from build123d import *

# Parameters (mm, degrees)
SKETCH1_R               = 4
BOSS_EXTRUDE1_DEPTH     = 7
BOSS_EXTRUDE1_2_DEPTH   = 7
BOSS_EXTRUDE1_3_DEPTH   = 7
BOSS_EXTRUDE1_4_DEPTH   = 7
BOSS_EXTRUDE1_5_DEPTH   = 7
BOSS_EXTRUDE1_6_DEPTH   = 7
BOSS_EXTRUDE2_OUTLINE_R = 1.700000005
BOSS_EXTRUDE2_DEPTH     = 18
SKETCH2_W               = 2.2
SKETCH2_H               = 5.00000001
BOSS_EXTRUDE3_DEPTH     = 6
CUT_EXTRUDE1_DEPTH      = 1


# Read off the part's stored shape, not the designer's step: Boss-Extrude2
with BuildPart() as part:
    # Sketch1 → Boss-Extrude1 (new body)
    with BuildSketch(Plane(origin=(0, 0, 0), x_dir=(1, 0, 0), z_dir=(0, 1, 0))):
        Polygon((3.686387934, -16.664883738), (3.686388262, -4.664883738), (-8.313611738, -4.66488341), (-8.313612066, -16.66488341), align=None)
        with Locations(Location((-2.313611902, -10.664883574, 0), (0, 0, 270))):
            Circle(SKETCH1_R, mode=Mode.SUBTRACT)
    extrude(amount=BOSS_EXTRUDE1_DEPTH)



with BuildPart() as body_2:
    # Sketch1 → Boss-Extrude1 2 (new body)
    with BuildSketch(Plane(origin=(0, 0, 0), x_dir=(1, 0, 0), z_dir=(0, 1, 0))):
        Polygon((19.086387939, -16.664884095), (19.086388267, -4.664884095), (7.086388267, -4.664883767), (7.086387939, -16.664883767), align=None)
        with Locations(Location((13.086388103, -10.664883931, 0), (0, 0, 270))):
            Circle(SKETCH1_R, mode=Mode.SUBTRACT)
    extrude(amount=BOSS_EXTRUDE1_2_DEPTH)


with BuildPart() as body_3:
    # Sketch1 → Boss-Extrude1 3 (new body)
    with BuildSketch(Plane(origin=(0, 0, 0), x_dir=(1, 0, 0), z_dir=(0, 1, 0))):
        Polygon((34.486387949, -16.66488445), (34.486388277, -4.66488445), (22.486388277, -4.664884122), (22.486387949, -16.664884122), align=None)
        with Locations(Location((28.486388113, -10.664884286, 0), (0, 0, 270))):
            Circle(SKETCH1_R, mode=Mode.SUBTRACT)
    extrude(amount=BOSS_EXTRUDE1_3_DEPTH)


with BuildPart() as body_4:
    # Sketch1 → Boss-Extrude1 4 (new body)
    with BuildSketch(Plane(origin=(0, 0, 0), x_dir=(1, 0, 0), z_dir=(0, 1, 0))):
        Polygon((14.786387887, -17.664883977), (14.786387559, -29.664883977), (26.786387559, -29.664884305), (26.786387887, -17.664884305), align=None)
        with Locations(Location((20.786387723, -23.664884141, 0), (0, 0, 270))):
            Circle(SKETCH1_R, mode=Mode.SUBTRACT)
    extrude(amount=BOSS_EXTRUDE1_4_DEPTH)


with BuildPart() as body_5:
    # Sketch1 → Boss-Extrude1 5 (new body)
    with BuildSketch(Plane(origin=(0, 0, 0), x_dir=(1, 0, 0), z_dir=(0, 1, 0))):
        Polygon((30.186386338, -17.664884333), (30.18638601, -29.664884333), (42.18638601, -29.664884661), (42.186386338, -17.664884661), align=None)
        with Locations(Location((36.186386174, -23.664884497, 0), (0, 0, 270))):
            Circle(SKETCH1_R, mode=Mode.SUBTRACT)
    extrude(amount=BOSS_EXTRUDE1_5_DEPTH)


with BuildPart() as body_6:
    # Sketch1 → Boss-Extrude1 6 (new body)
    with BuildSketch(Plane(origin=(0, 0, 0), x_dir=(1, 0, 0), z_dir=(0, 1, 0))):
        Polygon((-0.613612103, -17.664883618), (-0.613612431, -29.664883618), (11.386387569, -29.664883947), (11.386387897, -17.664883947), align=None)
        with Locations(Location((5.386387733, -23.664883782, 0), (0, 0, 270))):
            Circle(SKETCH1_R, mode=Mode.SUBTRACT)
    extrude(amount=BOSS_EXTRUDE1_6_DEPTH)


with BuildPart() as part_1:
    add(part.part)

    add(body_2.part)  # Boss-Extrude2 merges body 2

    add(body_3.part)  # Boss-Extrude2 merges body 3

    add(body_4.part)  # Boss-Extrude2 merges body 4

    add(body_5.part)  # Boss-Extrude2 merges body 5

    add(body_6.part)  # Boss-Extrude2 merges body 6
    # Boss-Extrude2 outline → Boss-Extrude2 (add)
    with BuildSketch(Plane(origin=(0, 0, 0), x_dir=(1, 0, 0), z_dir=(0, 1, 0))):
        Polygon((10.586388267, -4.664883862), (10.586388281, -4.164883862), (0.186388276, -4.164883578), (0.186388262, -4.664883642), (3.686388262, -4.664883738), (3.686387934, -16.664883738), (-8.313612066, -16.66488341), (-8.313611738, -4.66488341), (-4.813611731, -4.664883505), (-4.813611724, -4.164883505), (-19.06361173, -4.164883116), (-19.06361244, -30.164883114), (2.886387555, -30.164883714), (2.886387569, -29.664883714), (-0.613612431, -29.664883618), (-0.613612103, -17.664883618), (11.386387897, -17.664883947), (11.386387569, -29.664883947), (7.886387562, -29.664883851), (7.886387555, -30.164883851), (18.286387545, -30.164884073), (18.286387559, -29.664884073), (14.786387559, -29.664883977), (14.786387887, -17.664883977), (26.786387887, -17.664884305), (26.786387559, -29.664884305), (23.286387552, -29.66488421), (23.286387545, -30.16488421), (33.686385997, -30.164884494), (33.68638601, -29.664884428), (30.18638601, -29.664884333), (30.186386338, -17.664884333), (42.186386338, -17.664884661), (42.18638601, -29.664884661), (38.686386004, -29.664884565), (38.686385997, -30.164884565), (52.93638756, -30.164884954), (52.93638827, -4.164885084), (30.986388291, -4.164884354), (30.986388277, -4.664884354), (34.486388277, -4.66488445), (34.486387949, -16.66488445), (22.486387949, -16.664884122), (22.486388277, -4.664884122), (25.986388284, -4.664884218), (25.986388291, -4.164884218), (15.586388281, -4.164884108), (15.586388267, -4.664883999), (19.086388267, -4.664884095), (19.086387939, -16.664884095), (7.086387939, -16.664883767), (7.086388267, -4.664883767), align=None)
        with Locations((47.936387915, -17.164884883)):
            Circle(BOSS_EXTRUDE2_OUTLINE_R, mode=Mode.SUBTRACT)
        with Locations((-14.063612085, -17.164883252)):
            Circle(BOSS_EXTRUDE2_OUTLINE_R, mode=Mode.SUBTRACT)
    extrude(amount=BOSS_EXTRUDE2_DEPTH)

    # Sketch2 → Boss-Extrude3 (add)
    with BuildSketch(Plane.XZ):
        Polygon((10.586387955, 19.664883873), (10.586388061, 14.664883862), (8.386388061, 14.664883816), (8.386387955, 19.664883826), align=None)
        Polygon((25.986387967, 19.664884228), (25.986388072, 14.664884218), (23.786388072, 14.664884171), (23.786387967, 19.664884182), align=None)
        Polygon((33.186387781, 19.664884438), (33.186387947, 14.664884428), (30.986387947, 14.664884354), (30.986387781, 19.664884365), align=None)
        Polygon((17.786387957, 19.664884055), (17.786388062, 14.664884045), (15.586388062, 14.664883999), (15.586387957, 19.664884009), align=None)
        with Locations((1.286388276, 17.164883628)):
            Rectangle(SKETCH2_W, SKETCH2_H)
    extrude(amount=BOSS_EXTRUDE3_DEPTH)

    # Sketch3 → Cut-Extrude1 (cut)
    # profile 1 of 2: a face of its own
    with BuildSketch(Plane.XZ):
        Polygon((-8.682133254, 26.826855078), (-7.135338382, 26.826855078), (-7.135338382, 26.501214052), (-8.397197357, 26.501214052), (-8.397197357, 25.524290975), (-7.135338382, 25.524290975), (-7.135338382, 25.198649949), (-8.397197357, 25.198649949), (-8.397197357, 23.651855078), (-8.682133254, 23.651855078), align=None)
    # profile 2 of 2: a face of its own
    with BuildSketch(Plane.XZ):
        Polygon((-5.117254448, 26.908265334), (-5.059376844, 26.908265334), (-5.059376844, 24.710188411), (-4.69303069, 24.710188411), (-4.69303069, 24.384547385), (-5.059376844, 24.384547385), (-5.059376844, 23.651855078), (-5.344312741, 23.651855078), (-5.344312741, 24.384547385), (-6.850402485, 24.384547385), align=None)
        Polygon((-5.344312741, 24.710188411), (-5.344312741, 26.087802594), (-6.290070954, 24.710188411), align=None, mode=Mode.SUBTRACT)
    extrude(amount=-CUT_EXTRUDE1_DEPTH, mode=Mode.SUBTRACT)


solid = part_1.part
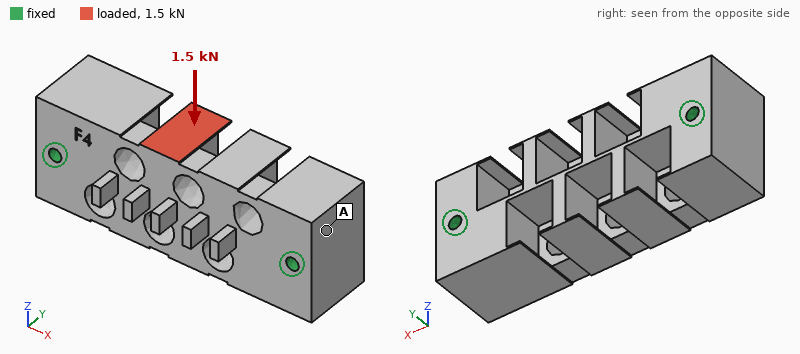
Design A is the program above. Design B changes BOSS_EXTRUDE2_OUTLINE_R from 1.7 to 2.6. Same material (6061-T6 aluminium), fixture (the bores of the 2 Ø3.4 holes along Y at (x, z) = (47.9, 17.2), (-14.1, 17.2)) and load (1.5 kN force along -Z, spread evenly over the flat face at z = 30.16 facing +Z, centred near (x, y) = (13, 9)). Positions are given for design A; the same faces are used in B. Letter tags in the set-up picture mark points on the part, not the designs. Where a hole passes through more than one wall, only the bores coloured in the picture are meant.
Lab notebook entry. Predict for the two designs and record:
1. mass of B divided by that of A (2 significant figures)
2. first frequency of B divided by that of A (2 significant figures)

0.98
1.1
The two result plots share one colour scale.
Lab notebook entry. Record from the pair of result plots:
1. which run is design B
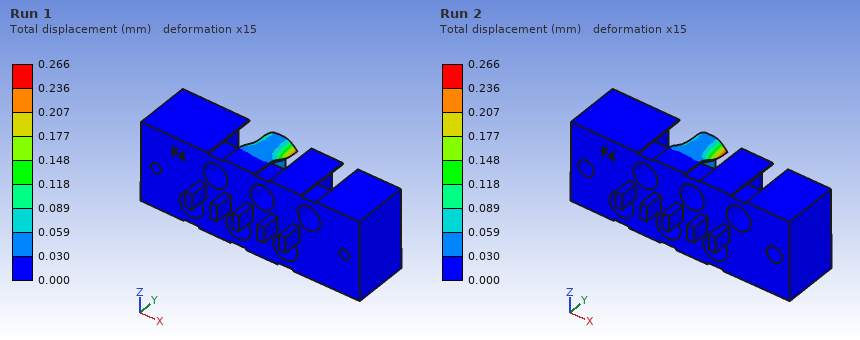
Run 2
